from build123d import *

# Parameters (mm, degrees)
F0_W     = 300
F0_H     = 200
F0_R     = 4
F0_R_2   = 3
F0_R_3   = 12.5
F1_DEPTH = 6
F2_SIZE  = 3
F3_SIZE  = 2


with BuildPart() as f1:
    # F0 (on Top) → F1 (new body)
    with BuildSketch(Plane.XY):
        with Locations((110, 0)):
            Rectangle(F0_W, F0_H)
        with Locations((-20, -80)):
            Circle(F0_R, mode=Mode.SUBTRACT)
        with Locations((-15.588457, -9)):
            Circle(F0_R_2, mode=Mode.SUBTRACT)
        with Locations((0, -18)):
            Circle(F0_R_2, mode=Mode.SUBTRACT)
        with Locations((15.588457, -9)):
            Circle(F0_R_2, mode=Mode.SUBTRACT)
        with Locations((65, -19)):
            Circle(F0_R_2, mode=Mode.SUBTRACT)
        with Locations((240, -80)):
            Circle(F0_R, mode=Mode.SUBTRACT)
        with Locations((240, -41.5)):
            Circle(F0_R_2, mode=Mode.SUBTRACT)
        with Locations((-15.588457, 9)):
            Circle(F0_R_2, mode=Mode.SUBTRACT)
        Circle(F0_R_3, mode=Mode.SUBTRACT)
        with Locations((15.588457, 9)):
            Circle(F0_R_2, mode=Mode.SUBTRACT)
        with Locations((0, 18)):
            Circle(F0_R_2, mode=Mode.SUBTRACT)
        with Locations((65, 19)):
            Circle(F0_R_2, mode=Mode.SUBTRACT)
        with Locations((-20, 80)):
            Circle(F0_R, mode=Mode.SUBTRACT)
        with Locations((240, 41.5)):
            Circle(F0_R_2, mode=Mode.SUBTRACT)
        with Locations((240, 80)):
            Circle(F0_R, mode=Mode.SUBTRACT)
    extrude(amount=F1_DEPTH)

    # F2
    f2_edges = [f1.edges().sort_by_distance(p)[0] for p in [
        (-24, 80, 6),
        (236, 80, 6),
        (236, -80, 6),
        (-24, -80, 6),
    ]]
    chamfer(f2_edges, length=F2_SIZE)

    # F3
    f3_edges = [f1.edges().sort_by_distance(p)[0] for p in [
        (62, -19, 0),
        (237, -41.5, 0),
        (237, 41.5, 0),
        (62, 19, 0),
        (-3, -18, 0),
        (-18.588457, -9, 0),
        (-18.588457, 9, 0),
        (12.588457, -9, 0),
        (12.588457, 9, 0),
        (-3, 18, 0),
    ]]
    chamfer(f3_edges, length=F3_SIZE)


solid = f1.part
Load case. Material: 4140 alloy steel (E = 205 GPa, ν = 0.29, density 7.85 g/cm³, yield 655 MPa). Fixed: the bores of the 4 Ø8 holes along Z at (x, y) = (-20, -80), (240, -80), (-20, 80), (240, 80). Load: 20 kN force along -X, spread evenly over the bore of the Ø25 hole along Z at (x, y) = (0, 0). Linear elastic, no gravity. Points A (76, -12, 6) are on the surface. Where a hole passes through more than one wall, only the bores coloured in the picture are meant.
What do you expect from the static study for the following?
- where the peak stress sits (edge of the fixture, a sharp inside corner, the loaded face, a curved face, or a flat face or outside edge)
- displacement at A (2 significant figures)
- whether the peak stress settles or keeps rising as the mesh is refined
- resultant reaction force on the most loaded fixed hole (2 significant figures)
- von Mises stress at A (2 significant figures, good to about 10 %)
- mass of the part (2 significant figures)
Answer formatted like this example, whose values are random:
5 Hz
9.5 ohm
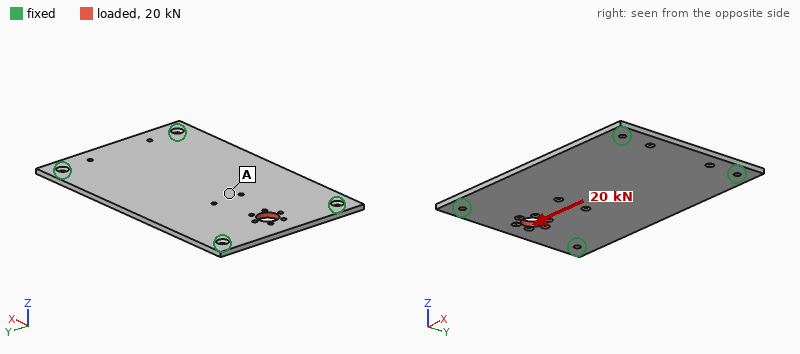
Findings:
edge of the fixture
13 µm
keeps rising
6.6 kN
22 MPa
2.8 kg
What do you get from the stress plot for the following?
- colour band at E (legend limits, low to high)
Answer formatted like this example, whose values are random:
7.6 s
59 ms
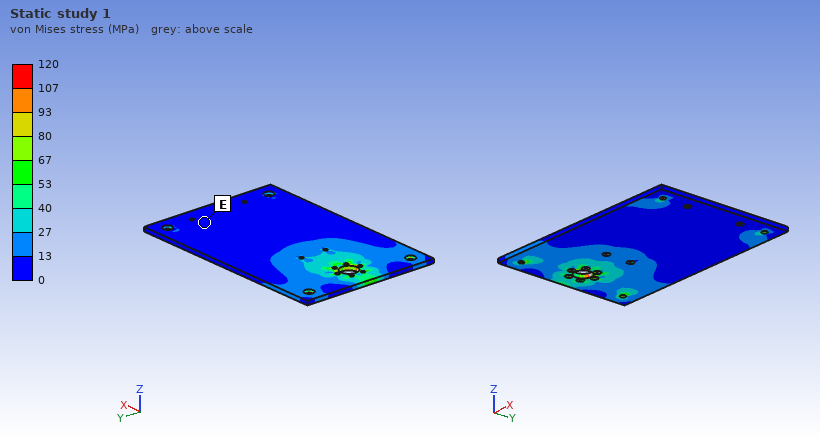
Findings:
0 to 13 MPa
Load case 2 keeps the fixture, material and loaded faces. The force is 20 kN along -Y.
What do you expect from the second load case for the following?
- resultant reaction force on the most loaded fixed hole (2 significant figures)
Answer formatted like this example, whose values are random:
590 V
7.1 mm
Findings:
8.9 kN
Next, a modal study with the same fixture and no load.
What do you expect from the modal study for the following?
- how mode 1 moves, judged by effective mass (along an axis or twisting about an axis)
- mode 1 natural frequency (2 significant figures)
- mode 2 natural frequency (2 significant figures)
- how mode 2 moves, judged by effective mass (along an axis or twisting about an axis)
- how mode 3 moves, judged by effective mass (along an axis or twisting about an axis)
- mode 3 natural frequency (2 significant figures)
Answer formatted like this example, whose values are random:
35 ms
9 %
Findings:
along Z
350 Hz
570 Hz
twisting about X
twisting about Y
900 Hz
